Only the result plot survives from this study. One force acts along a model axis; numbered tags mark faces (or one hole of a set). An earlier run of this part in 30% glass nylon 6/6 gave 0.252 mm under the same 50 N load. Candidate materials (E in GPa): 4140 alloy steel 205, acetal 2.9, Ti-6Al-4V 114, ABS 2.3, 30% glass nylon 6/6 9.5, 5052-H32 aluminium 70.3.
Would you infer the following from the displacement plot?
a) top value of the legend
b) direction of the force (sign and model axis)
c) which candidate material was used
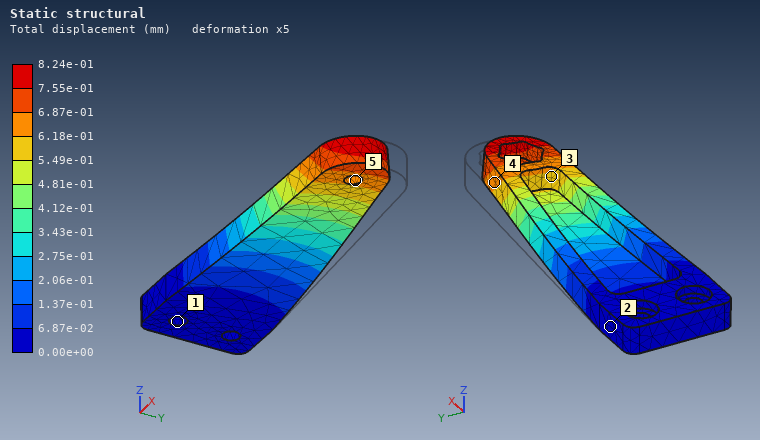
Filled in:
8.24e-01 mm
-Y
acetal
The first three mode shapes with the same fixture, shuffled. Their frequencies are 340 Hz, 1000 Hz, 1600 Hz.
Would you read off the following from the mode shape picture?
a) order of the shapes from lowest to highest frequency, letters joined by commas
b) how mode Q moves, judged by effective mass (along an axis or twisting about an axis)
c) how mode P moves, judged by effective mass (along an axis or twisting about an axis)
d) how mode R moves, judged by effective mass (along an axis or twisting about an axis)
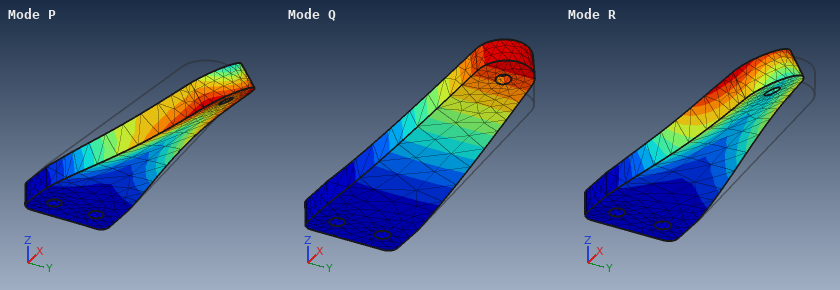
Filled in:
Q, R, P
along Z
along Y
along Y
